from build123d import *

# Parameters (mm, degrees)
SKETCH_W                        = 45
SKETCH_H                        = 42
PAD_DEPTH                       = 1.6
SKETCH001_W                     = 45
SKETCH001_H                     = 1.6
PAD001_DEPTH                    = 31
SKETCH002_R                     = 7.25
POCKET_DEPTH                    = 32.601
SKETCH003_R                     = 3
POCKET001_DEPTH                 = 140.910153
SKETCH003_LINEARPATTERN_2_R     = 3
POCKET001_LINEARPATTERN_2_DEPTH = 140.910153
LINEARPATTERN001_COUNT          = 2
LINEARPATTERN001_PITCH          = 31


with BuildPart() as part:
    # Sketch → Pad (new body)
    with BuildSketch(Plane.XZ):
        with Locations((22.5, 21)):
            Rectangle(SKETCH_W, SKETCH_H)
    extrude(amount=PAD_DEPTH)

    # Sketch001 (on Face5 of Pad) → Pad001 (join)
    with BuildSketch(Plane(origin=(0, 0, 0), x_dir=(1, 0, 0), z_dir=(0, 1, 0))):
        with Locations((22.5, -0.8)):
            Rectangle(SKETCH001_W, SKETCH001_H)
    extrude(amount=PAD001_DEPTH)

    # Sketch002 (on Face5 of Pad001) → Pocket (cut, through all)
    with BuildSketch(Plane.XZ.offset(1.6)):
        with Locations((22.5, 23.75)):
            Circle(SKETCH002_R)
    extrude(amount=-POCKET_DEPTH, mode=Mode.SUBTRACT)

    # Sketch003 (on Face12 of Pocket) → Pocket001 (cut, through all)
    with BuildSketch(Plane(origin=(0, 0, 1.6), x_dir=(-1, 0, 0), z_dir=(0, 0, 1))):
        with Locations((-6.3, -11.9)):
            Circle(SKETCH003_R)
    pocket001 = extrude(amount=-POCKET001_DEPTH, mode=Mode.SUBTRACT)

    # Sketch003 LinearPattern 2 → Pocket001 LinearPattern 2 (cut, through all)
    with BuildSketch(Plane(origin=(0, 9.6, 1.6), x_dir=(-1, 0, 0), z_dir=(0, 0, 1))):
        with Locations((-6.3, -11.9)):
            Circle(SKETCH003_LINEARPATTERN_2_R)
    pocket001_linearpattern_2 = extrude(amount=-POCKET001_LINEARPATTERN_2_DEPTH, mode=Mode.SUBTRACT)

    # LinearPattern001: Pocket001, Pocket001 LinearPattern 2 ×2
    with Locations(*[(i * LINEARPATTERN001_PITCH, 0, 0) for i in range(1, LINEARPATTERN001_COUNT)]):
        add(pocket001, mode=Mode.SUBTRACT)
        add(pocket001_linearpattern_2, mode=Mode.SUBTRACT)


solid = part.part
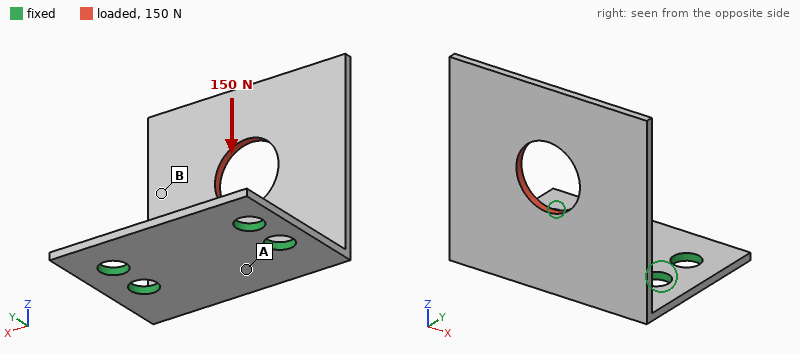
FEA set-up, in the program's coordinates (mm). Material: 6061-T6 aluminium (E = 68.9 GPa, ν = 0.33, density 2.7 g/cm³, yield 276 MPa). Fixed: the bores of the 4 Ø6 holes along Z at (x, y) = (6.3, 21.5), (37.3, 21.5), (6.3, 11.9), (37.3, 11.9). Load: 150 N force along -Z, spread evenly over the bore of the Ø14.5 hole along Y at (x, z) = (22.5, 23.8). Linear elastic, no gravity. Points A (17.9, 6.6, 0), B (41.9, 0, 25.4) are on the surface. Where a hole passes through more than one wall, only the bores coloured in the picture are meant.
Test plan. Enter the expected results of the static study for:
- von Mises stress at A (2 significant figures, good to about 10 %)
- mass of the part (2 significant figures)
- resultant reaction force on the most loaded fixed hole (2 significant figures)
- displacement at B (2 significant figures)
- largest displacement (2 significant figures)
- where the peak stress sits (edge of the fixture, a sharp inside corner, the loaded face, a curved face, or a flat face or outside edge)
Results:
30 MPa
13 g
91 N
0.22 mm
0.35 mm
a flat face or outside edge
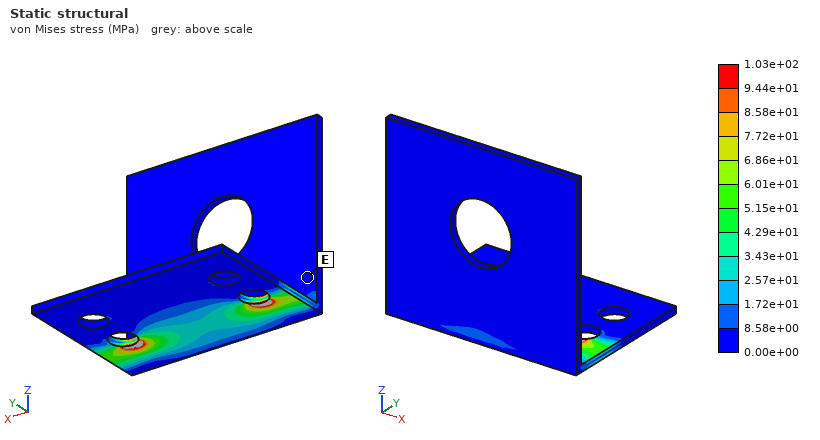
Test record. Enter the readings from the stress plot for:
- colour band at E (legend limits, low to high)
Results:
0.00e+00 to 8.58e+00 MPa
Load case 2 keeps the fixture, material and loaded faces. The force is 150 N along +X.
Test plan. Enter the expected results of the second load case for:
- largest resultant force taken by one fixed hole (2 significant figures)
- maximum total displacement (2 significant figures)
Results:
140 N
0.22 mm
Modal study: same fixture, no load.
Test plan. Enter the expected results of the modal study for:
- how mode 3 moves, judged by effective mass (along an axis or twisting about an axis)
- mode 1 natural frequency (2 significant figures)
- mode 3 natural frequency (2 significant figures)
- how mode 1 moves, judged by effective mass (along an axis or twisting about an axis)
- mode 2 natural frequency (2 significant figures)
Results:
along X
570 Hz
2200 Hz
along Y
1400 Hz
